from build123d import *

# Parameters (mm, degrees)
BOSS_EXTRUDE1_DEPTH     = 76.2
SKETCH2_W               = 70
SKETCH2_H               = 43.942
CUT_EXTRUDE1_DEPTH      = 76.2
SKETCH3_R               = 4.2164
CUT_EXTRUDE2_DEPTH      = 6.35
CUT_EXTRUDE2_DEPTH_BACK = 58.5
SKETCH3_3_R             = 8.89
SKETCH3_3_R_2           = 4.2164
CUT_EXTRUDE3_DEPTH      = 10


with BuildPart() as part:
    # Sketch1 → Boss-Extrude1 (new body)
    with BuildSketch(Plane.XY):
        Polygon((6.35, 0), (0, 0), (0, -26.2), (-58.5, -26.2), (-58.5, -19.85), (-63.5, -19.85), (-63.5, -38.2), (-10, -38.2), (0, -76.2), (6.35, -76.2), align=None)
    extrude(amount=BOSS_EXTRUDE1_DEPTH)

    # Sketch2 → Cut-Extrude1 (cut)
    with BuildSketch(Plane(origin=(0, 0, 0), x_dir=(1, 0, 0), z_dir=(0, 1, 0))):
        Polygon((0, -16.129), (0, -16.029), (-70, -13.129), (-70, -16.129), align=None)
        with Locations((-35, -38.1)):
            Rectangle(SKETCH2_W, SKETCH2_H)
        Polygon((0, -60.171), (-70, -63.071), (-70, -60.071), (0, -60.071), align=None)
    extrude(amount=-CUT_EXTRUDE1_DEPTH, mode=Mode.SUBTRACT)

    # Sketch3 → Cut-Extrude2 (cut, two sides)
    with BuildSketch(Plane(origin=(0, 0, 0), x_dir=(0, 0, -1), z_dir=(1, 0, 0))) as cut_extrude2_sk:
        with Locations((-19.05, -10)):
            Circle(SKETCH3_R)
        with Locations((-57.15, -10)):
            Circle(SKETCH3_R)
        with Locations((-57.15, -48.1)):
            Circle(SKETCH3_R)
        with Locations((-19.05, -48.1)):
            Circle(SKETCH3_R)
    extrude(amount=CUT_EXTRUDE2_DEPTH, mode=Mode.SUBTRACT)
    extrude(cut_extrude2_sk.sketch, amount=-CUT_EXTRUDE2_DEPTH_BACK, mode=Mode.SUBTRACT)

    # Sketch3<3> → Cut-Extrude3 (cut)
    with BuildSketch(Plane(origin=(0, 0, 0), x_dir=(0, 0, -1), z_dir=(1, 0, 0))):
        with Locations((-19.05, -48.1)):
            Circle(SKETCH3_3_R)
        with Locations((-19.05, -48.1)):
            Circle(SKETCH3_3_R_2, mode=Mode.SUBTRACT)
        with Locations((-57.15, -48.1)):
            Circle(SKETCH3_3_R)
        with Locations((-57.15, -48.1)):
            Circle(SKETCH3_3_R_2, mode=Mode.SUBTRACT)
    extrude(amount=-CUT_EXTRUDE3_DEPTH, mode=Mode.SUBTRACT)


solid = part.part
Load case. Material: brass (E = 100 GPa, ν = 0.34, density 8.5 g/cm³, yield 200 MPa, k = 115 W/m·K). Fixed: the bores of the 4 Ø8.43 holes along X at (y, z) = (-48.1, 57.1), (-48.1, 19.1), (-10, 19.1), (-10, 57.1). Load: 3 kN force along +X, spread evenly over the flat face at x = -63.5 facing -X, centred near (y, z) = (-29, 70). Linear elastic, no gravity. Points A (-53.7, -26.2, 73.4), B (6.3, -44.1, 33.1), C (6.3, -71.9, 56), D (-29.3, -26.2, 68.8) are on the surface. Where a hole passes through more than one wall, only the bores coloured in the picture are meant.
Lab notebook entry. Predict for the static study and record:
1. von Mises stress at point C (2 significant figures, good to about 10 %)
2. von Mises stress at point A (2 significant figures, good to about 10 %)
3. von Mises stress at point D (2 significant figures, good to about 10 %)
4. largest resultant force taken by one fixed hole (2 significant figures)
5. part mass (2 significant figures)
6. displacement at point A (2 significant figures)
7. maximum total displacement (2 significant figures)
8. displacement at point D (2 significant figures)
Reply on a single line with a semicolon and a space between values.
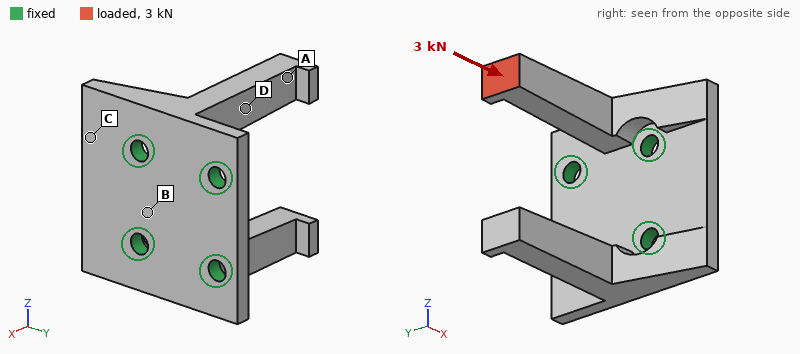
15 MPa; 51 MPa; 44 MPa; 1.6 kN; 540 g; 0.17 mm; 0.22 mm; 0.085 mm
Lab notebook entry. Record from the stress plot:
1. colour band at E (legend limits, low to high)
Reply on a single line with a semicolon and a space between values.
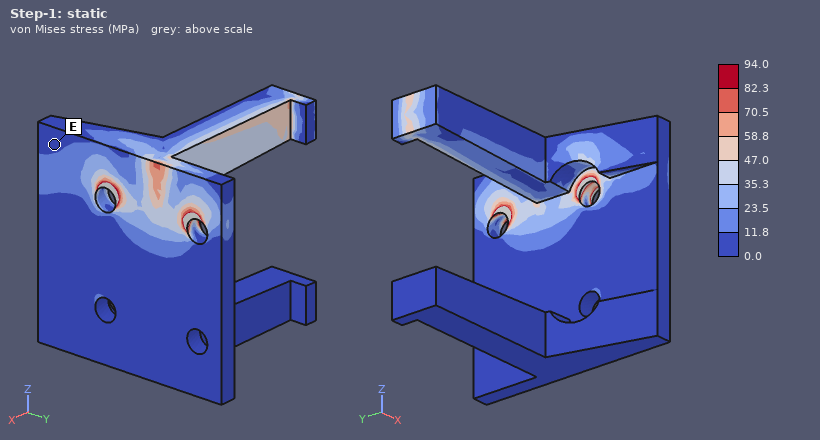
0.0 to 11.8 MPa
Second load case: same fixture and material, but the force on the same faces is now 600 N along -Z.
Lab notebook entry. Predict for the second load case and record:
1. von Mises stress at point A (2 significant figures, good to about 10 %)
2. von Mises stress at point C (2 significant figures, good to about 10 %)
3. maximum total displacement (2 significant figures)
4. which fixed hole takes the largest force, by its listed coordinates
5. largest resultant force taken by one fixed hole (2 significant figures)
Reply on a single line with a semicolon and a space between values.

16 MPa; 24 MPa; 0.33 mm; (-48.1, 57.1); 310 N
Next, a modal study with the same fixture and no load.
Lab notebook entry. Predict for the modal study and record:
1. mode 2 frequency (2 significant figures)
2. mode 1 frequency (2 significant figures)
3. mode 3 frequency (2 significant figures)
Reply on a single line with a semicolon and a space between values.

1200 Hz; 1200 Hz; 1500 Hz
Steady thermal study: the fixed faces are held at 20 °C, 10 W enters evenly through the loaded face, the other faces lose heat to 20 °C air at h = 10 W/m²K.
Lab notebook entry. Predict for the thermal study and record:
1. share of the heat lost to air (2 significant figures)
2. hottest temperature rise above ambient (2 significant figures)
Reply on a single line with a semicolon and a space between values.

7.0 %; 34 K
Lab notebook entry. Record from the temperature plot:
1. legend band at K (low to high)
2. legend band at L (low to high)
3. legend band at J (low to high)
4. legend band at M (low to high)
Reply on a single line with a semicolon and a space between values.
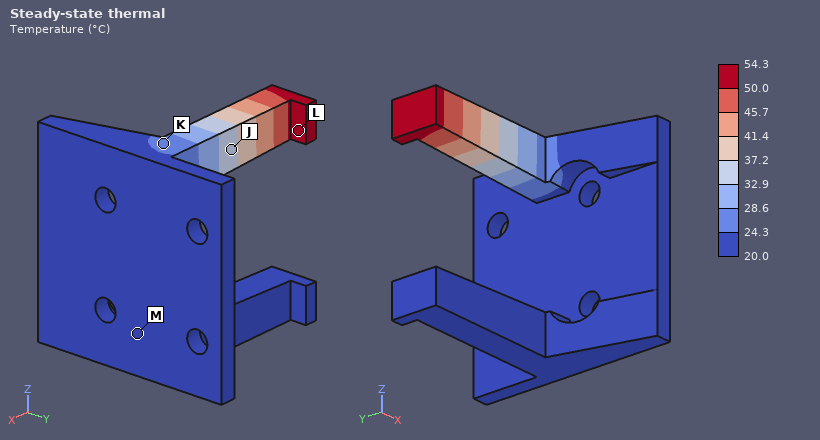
24.3 to 28.6 °C; 50.0 to 54.3 °C; 32.9 to 37.2 °C; 20.0 to 24.3 °C
